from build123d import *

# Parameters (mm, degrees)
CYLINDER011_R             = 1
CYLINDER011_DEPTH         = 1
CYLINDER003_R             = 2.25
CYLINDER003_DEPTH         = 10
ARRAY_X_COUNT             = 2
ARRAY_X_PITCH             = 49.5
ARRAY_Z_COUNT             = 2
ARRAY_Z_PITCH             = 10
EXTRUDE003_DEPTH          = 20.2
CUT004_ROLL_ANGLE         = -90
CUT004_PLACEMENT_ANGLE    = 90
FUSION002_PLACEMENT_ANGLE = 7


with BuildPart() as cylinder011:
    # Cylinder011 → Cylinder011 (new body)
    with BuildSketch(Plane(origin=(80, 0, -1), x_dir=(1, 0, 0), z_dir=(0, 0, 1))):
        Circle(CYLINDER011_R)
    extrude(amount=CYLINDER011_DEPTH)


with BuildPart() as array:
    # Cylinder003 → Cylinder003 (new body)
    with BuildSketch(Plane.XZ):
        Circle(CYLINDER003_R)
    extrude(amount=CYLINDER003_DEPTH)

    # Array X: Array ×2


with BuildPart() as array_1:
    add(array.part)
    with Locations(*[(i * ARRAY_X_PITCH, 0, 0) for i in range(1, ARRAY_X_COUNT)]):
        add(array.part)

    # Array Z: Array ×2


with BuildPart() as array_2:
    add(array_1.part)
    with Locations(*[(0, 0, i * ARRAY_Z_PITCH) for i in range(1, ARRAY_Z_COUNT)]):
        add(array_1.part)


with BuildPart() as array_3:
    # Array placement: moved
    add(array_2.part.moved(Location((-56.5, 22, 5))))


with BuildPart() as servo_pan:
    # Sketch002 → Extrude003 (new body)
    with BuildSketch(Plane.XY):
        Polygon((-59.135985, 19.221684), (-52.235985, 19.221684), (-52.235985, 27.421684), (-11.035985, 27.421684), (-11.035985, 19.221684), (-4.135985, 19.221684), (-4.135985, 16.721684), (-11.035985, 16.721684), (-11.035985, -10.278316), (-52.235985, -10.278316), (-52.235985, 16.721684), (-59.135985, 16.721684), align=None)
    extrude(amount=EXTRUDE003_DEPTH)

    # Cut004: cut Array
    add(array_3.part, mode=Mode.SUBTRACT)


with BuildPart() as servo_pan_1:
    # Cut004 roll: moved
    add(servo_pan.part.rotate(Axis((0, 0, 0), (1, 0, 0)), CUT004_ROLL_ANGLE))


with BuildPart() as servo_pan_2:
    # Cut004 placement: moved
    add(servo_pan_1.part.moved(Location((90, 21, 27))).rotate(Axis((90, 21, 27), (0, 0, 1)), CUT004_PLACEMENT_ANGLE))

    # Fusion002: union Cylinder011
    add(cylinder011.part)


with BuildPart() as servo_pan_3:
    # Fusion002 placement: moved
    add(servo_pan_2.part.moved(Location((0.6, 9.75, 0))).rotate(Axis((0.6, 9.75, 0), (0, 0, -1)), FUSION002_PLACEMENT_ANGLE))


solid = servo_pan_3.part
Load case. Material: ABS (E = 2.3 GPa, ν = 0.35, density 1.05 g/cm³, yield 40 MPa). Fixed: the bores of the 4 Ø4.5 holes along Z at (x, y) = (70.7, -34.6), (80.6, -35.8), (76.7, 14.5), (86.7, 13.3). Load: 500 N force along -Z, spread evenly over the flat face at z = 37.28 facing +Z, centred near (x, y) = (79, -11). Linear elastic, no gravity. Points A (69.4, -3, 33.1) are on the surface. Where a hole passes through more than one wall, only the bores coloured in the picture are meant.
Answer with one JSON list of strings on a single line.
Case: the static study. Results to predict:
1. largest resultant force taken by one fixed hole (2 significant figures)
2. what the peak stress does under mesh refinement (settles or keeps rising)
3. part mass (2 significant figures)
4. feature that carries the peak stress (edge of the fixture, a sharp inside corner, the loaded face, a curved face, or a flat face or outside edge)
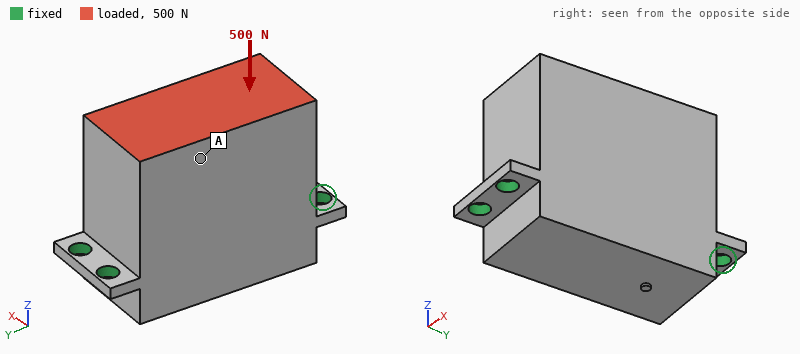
["130 N", "keeps rising", "34 g", "edge of the fixture"]
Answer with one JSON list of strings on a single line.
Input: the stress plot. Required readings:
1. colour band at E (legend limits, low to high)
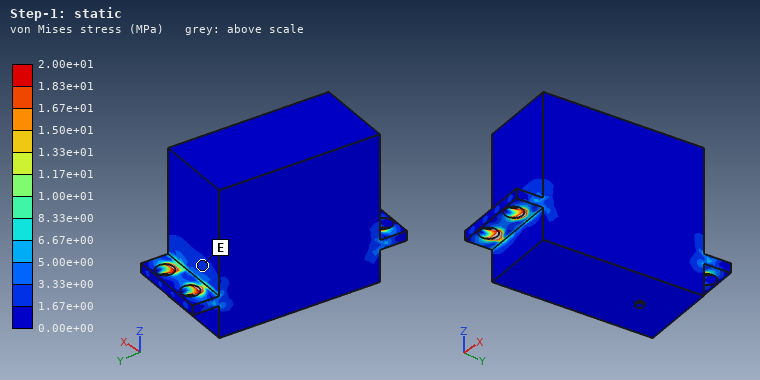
["1.67e+00 to 3.33e+00 MPa"]
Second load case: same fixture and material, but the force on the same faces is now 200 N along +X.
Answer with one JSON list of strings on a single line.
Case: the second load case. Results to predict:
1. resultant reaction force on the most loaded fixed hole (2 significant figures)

["250 N"]
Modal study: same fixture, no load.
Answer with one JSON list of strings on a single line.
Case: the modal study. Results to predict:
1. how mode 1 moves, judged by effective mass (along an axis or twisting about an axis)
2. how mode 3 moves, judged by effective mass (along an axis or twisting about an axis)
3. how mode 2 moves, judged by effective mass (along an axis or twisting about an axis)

["along X", "along Y", "along Z"]
